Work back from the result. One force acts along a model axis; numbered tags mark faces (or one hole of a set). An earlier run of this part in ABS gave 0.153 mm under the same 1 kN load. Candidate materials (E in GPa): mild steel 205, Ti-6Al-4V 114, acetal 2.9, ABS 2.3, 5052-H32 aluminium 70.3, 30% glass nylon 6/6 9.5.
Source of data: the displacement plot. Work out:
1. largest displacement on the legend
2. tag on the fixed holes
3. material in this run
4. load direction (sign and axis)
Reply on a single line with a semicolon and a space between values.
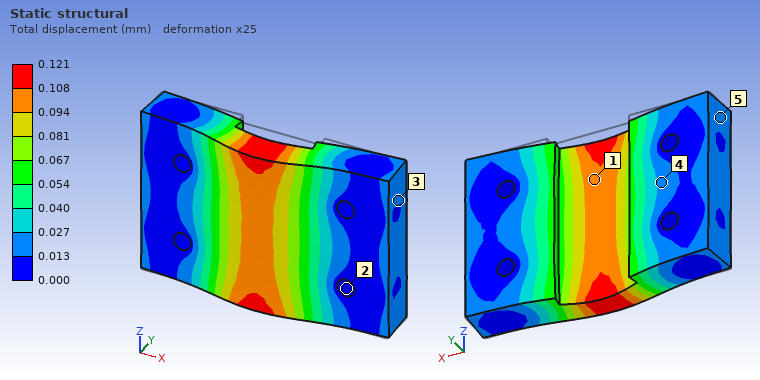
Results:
0.121 mm; 2; acetal; -Y
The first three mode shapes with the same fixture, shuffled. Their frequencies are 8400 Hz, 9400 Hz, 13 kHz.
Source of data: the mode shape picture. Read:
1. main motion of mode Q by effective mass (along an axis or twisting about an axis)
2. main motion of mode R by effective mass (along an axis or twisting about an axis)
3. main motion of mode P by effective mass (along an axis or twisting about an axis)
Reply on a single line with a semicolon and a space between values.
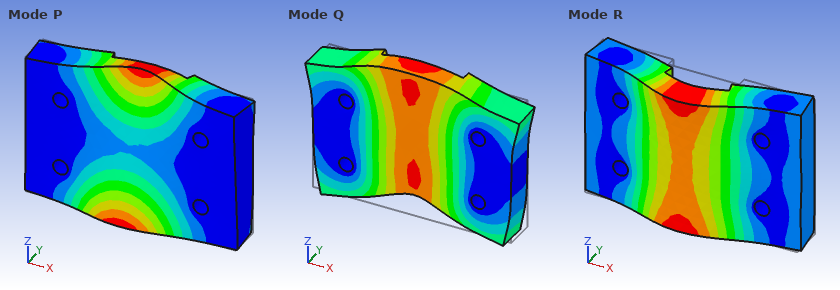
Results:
along Z; along Y; twisting about X
